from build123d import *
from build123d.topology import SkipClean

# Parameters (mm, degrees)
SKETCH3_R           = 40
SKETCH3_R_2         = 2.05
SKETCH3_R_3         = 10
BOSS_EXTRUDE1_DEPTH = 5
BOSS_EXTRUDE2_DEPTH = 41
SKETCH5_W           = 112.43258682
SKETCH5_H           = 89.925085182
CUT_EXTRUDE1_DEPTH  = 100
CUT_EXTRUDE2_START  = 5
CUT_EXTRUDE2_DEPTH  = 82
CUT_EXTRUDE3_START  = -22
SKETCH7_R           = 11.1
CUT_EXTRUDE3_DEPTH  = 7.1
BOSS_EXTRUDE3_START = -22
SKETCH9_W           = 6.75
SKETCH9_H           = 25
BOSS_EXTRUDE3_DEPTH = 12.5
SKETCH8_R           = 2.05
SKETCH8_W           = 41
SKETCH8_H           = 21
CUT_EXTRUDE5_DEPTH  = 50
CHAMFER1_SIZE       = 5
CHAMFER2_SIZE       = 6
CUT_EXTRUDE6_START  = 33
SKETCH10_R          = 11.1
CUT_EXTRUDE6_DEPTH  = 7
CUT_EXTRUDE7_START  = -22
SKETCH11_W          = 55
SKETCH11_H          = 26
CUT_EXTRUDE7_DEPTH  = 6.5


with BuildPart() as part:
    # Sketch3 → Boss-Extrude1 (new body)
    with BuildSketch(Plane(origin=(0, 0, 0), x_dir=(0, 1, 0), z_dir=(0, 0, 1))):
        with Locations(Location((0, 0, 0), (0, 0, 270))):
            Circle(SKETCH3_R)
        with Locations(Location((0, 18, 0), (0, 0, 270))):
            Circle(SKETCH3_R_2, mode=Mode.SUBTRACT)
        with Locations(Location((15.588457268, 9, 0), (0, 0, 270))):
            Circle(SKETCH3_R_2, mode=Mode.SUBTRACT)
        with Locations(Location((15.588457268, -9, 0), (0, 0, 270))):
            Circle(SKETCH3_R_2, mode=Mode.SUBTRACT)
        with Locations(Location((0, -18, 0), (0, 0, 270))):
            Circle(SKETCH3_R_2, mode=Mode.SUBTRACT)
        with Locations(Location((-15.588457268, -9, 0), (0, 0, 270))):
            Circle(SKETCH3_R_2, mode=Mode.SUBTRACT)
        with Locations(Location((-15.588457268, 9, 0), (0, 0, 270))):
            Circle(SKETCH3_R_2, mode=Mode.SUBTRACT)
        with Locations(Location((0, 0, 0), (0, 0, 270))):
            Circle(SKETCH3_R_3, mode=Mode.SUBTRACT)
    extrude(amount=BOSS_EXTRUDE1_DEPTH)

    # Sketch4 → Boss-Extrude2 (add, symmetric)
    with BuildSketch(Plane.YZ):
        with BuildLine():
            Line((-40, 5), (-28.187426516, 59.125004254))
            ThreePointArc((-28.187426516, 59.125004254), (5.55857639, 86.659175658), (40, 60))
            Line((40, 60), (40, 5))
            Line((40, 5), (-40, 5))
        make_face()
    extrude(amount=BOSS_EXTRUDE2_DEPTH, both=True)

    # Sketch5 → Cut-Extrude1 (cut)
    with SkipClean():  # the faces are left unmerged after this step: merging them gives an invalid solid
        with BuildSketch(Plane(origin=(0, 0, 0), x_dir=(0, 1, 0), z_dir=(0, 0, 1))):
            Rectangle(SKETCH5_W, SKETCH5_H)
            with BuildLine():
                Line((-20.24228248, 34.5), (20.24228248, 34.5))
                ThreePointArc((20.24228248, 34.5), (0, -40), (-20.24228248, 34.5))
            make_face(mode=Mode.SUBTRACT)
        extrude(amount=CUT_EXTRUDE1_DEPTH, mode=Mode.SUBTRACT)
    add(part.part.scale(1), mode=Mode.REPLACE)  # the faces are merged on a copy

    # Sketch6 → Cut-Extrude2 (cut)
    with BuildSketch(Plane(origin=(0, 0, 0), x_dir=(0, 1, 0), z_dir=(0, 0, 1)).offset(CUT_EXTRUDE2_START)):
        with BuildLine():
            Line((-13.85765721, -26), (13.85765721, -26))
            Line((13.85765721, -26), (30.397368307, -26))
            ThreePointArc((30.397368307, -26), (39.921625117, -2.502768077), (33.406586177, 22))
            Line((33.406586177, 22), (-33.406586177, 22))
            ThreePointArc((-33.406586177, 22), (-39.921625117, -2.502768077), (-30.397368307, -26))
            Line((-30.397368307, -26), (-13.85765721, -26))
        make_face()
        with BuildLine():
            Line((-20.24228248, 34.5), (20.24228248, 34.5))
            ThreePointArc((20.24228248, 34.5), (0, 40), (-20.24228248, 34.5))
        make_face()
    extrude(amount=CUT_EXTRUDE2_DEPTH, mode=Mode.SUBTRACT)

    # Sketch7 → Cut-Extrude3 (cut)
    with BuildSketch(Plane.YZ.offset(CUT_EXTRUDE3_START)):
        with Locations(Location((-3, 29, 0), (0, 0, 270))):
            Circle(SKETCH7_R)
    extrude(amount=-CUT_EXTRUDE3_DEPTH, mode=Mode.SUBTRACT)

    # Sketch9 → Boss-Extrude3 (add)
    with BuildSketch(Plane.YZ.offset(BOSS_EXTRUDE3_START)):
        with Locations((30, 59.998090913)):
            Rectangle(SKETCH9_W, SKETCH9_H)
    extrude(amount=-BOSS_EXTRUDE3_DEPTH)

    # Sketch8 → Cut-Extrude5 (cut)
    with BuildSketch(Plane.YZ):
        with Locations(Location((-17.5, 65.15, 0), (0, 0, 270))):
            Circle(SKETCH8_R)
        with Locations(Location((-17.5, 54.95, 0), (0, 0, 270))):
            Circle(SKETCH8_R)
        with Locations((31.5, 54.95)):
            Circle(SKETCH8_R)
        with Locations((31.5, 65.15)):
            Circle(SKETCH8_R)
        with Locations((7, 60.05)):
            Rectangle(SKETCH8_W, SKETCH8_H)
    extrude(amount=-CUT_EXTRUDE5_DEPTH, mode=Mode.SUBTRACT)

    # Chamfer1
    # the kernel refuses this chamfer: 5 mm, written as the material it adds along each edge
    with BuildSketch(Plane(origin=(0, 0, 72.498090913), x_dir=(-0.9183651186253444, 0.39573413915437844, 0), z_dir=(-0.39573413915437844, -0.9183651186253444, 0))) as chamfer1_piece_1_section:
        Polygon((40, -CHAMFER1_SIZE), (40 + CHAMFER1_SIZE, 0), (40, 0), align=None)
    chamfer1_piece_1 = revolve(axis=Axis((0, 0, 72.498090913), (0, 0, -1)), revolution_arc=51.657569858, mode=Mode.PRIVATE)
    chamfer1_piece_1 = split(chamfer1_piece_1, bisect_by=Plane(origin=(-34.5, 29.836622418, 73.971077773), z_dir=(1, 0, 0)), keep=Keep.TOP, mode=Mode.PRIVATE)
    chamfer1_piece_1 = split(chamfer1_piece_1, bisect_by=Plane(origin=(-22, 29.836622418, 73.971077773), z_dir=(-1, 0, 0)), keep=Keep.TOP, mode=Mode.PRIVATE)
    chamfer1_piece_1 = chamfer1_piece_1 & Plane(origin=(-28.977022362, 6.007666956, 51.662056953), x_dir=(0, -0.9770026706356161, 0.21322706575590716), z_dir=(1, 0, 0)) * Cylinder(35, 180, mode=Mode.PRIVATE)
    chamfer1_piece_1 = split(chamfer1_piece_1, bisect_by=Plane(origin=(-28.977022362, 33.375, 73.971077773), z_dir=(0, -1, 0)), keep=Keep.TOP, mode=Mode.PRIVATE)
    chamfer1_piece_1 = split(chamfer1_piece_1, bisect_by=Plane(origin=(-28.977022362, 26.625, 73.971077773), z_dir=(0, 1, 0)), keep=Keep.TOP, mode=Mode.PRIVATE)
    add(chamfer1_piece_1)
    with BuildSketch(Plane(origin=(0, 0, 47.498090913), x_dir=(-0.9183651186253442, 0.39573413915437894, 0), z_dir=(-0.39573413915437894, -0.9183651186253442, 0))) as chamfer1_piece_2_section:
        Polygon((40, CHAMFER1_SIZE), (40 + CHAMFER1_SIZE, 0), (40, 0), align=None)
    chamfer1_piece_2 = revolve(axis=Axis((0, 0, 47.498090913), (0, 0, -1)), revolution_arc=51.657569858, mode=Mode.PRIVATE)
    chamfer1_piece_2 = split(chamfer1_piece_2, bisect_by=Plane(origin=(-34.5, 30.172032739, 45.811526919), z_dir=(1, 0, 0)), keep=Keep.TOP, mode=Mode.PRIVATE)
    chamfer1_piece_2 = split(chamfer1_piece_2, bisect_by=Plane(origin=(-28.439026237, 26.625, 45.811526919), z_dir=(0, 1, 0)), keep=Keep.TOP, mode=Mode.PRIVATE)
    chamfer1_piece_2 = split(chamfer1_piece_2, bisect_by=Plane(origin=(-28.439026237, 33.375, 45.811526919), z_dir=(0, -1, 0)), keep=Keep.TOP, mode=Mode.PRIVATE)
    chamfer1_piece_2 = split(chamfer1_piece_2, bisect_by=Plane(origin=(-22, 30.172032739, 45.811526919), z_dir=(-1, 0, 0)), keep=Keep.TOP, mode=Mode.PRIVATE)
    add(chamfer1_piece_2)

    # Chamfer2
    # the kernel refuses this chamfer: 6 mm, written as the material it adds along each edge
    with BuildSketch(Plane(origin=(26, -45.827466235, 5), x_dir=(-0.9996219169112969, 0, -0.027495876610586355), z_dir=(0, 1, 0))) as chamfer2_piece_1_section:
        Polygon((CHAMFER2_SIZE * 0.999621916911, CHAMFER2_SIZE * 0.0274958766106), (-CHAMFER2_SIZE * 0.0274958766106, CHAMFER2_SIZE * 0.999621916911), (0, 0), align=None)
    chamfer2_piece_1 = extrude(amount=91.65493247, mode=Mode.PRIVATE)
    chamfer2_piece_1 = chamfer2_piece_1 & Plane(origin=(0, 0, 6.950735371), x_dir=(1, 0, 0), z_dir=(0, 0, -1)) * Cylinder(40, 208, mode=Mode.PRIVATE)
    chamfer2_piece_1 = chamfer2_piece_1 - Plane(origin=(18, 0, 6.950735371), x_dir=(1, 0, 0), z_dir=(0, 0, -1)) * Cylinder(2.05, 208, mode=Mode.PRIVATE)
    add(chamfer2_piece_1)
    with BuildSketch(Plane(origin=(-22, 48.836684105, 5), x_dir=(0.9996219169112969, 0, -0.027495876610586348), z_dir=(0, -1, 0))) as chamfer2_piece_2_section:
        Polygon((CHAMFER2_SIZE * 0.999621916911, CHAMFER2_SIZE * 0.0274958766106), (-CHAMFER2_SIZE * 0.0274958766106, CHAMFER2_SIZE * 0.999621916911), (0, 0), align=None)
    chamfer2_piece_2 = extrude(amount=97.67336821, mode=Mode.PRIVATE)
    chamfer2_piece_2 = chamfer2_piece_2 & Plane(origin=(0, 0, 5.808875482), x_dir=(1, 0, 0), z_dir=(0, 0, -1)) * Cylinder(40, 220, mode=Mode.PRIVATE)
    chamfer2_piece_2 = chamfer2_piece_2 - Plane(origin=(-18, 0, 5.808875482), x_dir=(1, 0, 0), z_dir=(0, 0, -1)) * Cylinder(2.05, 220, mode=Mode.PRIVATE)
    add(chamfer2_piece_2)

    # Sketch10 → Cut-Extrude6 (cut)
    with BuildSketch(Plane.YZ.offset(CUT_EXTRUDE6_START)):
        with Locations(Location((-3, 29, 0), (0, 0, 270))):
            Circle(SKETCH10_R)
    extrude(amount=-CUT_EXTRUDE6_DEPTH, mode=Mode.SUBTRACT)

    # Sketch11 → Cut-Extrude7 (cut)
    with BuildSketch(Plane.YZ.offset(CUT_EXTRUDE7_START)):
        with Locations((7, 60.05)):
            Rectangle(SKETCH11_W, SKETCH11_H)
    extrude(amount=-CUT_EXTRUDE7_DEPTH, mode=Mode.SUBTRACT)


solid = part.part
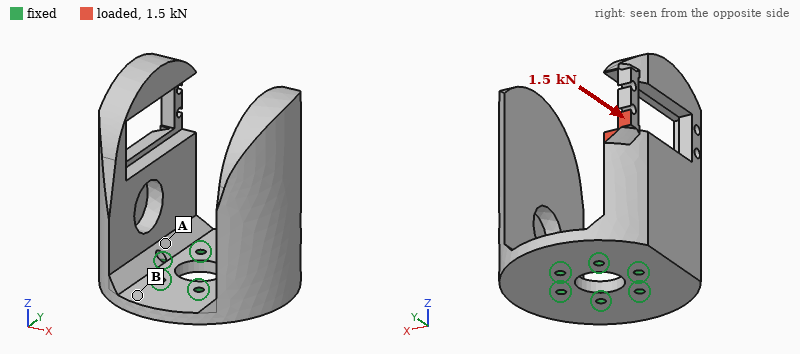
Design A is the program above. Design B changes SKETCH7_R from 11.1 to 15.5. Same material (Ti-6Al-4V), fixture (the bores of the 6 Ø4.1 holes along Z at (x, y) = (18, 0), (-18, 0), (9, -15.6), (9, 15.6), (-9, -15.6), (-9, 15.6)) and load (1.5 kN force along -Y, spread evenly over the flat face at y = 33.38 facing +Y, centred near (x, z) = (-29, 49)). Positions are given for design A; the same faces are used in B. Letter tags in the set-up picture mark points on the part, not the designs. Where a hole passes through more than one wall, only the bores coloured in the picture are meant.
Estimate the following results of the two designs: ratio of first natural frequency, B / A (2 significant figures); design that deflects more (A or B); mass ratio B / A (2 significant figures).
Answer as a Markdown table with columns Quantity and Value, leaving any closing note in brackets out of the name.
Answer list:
| Quantity | Value |
|---|---|
| ratio of first natural frequency, B / A | 1.0 |
| design that deflects more | B |
| mass ratio B / A | 0.98 |
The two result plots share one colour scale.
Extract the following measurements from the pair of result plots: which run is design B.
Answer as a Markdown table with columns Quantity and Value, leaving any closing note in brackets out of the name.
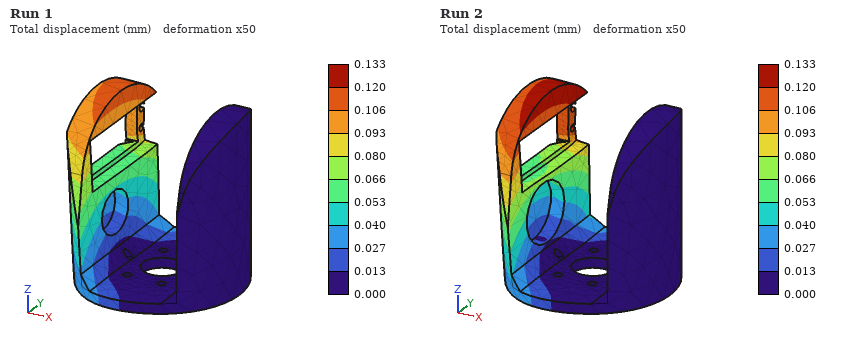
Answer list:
| Quantity | Value |
|---|---|
| which run is design B | Run 2 |
